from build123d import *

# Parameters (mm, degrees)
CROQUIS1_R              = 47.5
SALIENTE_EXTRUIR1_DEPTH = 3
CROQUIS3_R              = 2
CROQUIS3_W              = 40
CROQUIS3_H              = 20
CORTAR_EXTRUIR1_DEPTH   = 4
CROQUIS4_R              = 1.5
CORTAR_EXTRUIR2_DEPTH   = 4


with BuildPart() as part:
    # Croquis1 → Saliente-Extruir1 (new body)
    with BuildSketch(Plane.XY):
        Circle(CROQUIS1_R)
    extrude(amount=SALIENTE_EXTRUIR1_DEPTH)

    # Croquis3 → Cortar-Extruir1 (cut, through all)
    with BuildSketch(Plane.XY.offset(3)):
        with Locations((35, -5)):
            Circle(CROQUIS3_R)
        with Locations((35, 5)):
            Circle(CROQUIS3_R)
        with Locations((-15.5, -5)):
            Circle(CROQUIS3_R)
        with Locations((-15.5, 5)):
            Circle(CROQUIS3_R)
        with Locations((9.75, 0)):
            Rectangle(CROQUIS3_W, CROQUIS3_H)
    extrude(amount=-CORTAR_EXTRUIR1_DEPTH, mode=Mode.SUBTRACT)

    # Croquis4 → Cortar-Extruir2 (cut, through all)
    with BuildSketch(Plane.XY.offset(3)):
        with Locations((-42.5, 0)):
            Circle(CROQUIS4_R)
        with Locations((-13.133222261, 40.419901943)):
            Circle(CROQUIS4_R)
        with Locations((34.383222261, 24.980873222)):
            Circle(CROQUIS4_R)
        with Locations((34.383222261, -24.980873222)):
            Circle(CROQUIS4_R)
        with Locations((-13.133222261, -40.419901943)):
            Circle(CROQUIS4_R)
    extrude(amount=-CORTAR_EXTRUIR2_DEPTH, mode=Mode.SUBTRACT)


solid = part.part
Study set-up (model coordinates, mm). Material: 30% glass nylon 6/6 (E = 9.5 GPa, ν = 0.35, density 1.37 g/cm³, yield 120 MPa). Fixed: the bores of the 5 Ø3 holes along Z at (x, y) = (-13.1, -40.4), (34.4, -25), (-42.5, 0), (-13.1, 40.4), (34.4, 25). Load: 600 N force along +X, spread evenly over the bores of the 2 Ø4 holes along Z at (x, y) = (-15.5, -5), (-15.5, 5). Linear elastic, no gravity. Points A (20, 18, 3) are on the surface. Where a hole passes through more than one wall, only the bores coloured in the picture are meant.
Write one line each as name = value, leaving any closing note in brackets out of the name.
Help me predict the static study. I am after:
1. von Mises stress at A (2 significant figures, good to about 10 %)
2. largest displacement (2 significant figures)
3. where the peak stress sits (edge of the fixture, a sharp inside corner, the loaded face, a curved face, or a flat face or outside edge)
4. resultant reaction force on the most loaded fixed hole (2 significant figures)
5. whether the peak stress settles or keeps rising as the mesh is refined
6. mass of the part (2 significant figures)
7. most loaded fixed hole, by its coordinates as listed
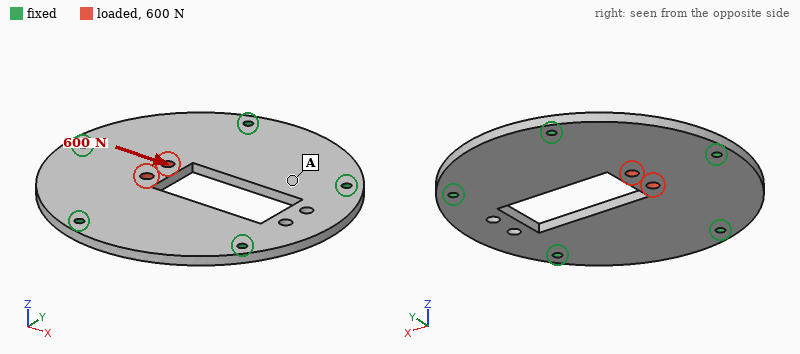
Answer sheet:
von Mises stress at A = 1.8 MPa
largest displacement = 27 µm
where the peak stress sits = edge of the fixture
resultant reaction force on the most loaded fixed hole = 310 N
whether the peak stress settles or keeps rising as the mesh is refined = keeps rising
mass of the part = 25 g
most loaded fixed hole, by its coordinates as listed = (-42.5, 0)
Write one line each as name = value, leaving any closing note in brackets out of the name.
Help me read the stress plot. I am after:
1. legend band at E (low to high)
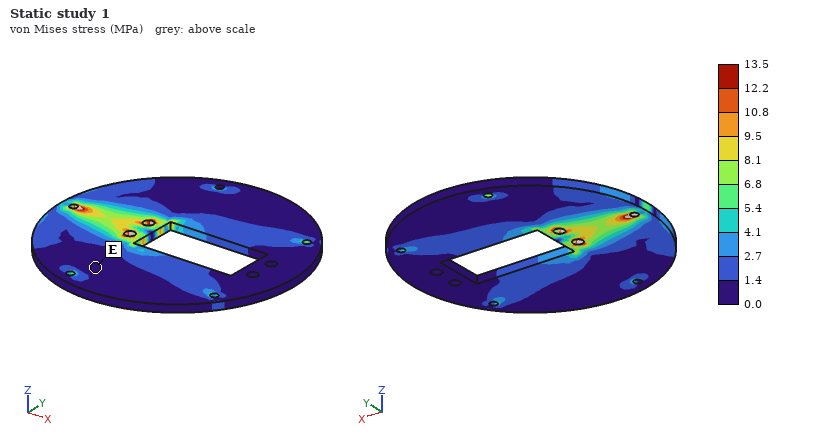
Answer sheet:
legend band at E = 0.0 to 1.4 MPa
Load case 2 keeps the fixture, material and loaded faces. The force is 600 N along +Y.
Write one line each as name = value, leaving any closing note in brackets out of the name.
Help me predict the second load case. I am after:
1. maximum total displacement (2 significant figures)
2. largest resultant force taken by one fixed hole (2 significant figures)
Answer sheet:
maximum total displacement = 26 µm
largest resultant force taken by one fixed hole = 210 N
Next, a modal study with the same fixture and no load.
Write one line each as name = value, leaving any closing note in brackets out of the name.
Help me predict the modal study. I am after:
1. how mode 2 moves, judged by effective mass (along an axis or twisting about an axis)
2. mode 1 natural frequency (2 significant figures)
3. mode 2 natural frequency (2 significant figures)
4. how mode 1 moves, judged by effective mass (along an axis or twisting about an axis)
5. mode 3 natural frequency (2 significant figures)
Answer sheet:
how mode 2 moves, judged by effective mass = twisting about X
mode 1 natural frequency = 1700 Hz
mode 2 natural frequency = 2500 Hz
how mode 1 moves, judged by effective mass = along Z
mode 3 natural frequency = 2700 Hz
